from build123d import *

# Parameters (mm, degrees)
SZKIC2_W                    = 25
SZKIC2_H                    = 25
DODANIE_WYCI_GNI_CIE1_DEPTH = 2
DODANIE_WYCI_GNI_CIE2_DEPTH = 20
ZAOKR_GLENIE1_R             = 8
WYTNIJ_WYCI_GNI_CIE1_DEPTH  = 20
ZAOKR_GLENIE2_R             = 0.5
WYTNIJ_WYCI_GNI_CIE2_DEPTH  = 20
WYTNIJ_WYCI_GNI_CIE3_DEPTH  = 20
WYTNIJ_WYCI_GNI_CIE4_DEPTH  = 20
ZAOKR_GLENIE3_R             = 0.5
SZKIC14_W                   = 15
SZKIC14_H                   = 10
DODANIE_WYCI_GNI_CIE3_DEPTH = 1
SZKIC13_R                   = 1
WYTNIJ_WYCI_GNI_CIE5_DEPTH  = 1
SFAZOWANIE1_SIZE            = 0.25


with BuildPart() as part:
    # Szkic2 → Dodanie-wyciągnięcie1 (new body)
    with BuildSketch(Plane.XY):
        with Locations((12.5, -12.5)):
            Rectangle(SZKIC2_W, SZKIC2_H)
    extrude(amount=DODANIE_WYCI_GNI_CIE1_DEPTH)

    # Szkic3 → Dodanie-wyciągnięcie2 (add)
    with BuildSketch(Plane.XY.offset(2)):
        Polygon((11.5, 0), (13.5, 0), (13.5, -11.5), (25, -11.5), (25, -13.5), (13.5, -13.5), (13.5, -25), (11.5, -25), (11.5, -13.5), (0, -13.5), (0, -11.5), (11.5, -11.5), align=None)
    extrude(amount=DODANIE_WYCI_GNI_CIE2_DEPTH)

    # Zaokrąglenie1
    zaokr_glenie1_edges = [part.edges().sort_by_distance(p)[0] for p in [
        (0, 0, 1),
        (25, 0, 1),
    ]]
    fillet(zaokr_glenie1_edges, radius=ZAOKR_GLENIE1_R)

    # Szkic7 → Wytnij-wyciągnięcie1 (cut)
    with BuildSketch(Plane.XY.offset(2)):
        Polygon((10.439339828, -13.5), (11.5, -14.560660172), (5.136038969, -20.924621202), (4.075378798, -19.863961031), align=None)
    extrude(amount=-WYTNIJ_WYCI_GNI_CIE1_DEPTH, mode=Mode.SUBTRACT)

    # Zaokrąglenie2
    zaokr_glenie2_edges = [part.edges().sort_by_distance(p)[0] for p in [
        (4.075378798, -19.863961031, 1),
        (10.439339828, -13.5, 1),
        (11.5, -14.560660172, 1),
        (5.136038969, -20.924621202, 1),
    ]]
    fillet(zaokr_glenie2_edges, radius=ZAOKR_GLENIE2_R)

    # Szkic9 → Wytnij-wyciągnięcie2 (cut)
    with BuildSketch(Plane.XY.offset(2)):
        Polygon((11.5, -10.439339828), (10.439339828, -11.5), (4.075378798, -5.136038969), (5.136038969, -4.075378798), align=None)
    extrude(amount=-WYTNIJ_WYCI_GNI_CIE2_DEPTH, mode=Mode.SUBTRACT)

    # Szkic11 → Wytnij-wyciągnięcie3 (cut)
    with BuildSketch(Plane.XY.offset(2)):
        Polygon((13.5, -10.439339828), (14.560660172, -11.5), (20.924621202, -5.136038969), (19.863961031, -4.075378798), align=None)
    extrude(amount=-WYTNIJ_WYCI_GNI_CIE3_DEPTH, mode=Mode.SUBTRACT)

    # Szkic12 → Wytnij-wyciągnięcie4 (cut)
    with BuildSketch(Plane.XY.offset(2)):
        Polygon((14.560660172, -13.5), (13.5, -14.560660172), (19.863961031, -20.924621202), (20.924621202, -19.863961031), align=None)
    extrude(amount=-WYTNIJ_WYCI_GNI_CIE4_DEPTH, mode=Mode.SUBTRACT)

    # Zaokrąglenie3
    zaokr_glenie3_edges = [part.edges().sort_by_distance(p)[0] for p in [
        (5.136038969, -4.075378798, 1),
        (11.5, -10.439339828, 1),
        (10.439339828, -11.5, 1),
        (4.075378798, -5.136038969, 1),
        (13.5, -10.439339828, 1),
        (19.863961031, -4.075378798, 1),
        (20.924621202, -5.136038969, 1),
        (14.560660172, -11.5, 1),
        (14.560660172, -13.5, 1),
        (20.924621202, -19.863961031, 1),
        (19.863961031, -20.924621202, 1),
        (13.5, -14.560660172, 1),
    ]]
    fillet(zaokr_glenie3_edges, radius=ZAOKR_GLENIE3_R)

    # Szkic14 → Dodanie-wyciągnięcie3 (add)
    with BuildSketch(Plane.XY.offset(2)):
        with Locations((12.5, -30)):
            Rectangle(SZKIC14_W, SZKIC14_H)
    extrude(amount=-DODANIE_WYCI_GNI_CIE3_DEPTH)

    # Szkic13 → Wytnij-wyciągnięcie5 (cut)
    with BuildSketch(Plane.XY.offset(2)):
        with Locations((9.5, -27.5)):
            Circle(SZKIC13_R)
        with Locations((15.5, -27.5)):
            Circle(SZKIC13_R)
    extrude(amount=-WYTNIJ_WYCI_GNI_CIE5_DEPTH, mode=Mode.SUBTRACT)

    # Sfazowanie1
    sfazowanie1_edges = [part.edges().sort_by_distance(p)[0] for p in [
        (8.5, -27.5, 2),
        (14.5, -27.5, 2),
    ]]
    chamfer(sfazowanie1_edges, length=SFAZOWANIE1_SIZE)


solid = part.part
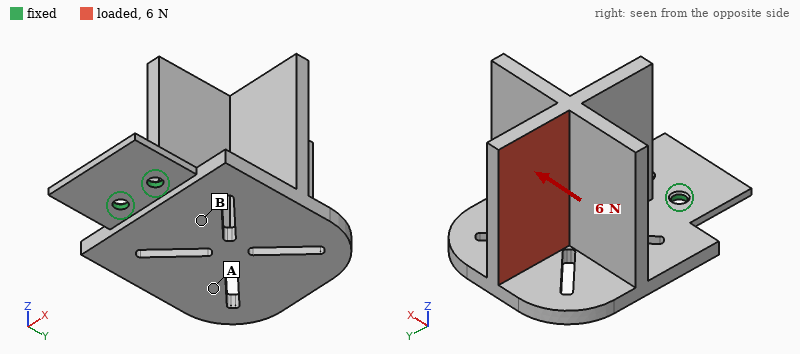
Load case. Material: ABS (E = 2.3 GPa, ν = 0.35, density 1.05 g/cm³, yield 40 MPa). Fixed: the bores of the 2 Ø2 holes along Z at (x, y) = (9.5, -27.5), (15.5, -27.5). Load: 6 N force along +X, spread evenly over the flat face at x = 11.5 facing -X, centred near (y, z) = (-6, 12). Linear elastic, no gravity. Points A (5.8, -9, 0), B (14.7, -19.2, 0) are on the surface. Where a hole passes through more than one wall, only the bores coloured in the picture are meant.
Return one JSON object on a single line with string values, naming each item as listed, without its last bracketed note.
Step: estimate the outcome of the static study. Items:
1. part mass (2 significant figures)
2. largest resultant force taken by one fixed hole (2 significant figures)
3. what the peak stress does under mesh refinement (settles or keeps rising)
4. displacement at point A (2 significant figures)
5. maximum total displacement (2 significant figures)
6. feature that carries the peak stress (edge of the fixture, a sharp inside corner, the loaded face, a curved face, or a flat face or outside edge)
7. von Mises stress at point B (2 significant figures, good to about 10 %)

{"part mass": "3.3 g", "largest resultant force taken by one fixed hole": "20 N", "what the peak stress does under mesh refinement": "keeps rising", "displacement at point A": "0.14 mm", "maximum total displacement": "0.56 mm", "feature that carries the peak stress": "edge of the fixture", "von Mises stress at point B": "2.4 MPa"}
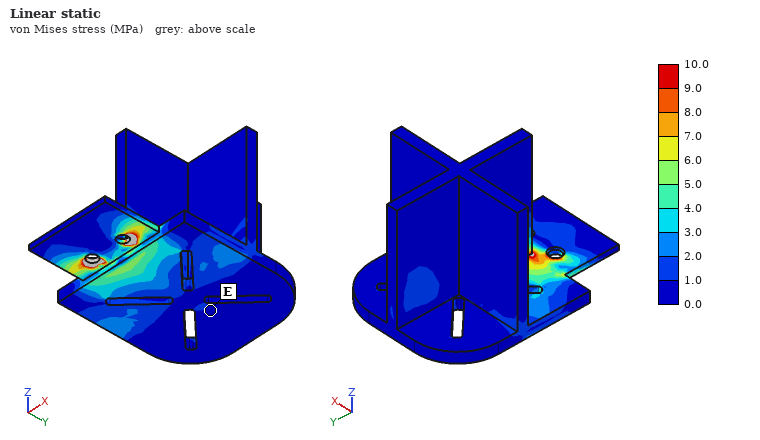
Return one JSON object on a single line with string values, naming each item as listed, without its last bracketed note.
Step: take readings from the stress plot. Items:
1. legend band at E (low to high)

{"legend band at E": "0.0 to 1.0 MPa"}
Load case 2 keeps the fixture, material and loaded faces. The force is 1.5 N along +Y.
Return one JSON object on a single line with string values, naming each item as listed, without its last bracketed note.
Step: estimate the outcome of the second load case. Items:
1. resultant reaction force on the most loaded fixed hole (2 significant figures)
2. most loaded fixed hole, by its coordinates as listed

{"resultant reaction force on the most loaded fixed hole": "1.0 N", "most loaded fixed hole, by its coordinates as listed": "(9.5, -27.5)"}
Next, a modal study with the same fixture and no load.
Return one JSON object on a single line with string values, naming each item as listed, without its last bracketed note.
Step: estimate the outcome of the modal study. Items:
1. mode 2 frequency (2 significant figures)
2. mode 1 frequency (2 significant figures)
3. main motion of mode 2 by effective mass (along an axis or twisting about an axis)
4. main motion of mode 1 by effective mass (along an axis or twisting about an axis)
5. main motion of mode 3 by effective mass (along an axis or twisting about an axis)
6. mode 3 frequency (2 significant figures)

{"mode 2 frequency": "450 Hz", "mode 1 frequency": "170 Hz", "main motion of mode 2 by effective mass": "along X", "main motion of mode 1 by effective mass": "along Z", "main motion of mode 3 by effective mass": "along X", "mode 3 frequency": "1500 Hz"}
